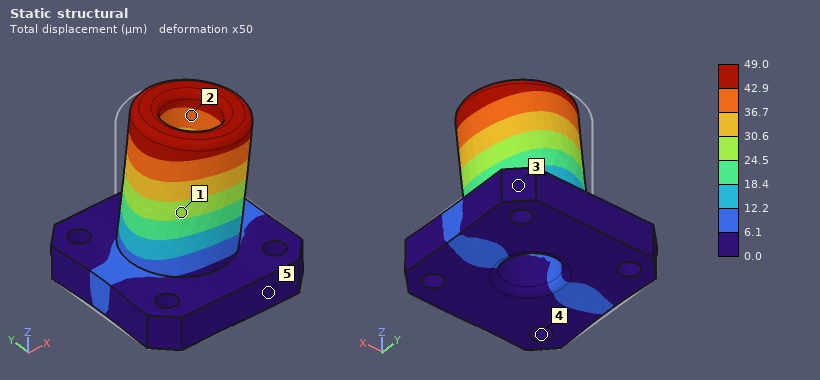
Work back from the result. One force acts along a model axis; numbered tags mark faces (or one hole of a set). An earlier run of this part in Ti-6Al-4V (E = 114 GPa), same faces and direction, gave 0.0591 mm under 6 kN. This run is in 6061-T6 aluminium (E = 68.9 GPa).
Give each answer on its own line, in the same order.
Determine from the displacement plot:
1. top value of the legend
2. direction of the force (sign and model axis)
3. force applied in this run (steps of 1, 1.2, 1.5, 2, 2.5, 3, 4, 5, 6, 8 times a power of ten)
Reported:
49.0 µm
+X
3 kN
